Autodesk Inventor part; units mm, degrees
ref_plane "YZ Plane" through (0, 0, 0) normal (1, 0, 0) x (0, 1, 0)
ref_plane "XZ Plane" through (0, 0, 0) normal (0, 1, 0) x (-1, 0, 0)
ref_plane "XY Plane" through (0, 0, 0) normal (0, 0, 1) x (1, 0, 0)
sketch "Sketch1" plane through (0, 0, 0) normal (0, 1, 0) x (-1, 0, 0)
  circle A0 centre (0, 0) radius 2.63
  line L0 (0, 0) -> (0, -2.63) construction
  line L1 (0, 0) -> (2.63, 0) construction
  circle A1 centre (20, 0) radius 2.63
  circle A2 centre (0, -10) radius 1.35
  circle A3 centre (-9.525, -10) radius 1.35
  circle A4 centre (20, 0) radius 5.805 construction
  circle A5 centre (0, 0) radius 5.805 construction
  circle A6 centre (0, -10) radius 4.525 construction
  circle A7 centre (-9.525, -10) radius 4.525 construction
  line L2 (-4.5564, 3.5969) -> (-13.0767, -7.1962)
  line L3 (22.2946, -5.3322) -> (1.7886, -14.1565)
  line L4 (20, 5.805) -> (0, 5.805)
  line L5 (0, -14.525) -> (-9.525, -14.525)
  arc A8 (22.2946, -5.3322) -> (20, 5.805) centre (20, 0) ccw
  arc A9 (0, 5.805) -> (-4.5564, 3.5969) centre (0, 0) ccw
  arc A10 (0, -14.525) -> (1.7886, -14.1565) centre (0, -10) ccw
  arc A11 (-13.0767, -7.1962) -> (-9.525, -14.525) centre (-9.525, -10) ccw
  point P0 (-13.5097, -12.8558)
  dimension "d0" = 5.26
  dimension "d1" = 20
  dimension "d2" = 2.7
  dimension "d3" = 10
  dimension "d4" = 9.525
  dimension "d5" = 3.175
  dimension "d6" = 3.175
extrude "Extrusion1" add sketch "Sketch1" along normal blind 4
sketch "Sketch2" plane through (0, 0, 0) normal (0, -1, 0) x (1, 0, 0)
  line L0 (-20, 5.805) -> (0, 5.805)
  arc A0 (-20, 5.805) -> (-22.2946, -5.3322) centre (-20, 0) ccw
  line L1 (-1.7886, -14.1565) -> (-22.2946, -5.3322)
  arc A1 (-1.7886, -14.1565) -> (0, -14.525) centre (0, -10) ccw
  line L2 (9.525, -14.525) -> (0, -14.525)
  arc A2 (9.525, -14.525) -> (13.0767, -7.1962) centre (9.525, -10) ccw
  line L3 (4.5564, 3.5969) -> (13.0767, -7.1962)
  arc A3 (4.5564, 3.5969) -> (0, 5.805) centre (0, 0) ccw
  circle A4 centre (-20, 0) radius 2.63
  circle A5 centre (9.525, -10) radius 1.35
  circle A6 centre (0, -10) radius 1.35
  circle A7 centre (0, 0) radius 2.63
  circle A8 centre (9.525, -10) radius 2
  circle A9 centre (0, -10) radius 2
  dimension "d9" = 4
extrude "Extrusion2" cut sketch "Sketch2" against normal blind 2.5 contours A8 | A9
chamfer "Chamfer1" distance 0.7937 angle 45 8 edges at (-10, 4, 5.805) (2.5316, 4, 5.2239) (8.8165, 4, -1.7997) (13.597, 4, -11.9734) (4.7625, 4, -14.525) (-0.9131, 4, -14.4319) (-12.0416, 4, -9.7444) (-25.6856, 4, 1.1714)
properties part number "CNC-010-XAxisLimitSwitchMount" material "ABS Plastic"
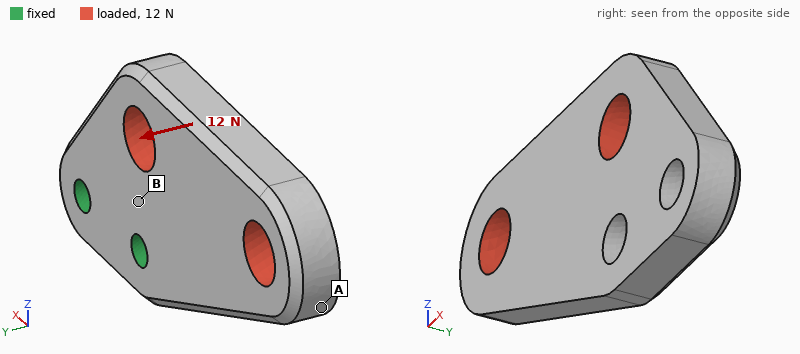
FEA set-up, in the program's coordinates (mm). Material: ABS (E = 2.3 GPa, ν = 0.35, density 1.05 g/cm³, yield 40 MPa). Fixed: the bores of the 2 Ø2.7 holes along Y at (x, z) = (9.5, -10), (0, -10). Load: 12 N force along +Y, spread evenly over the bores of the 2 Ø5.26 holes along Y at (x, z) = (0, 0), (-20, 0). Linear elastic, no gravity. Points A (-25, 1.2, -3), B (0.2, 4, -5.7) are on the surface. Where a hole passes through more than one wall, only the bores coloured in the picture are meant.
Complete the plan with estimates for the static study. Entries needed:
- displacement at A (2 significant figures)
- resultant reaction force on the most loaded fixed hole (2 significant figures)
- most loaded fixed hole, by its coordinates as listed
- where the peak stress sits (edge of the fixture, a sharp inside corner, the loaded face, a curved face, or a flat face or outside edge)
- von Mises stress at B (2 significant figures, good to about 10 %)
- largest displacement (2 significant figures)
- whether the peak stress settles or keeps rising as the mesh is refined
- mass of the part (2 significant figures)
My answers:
0.26 mm
23 N
(0, -10)
edge of the fixture
3.6 MPa
0.32 mm
keeps rising
2.1 g
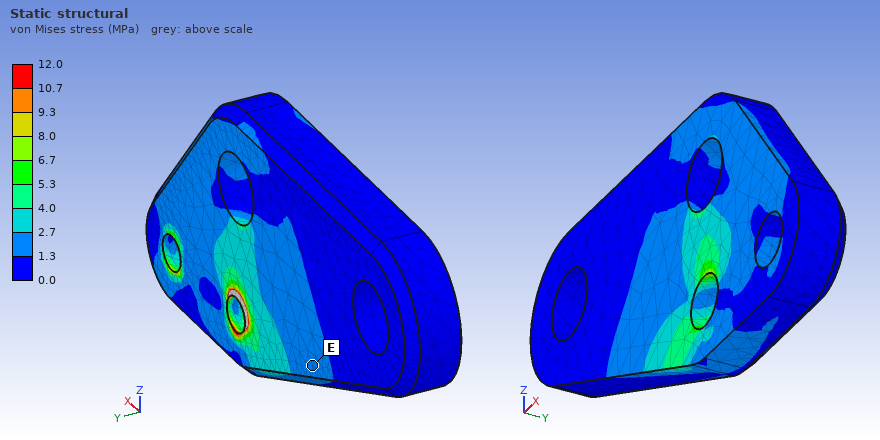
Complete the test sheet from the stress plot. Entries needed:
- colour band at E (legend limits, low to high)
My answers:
1.3 to 2.7 MPa
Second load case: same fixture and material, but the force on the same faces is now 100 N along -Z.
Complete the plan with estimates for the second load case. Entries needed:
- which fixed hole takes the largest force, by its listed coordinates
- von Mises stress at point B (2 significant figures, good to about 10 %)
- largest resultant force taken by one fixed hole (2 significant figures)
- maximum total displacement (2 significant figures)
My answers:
(0, -10)
8.3 MPa
180 N
0.33 mm
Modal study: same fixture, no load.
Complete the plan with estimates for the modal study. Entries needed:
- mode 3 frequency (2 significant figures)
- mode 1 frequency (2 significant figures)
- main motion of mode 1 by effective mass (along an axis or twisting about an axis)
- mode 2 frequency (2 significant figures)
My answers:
3100 Hz
1100 Hz
along Y
2800 Hz
